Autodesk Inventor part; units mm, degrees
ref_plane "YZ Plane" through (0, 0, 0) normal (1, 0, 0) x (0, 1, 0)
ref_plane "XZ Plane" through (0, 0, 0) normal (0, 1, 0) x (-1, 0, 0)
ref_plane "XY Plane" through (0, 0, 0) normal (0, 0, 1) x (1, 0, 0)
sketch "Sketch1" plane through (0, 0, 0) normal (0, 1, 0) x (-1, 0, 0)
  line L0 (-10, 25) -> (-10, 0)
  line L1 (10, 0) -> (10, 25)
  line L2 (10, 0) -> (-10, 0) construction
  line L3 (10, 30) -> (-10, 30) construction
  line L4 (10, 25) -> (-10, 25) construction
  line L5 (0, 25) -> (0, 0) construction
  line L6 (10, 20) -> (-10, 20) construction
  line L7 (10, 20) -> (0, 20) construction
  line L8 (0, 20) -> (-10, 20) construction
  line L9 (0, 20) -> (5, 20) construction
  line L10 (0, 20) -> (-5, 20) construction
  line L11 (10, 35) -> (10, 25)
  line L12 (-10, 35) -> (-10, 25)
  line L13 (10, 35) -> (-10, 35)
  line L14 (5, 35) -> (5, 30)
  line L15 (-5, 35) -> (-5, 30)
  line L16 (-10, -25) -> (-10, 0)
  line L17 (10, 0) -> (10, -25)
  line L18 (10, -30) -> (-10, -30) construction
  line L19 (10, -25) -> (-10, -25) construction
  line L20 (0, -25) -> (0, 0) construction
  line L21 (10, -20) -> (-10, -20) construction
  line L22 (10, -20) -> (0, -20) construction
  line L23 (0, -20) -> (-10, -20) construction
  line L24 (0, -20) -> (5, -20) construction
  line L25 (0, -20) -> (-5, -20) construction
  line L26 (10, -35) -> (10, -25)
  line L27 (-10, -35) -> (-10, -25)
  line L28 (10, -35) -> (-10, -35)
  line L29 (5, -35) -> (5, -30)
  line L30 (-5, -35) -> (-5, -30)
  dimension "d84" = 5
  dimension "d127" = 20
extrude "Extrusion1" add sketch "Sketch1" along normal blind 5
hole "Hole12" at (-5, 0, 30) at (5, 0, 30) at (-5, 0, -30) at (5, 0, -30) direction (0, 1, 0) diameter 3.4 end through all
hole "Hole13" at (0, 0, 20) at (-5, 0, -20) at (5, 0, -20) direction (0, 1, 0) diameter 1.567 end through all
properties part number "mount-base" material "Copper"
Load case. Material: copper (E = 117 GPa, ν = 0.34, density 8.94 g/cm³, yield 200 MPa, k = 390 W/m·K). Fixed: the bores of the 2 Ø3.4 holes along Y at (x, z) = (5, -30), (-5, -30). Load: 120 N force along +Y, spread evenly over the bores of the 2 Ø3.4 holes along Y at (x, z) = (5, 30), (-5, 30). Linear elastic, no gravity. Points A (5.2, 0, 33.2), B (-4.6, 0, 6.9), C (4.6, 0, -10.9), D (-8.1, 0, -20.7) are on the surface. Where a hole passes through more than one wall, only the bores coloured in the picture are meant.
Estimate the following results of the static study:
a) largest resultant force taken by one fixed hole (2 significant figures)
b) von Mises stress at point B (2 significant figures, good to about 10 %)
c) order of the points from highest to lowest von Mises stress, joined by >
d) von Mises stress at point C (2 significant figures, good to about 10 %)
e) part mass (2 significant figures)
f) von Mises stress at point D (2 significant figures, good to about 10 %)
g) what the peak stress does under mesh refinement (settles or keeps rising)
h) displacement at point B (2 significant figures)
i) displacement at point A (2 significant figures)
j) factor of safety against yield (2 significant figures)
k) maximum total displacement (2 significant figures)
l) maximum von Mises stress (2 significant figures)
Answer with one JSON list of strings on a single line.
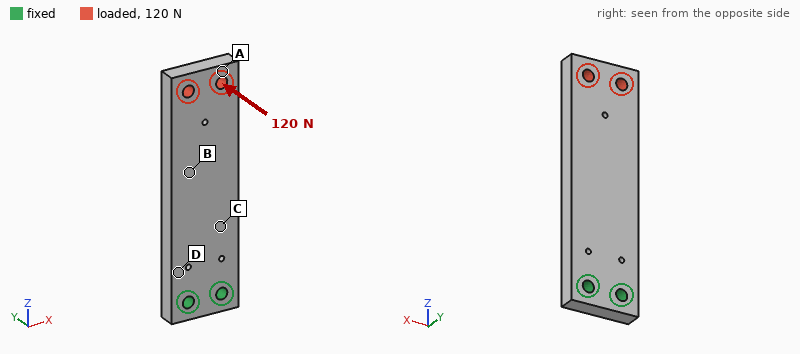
["60 N", "33 MPa", "D > C > B > A", "58 MPa", "61 g", "78 MPa", "settles", "0.16 mm", "0.38 mm", "1.2", "0.39 mm", "160 MPa"]
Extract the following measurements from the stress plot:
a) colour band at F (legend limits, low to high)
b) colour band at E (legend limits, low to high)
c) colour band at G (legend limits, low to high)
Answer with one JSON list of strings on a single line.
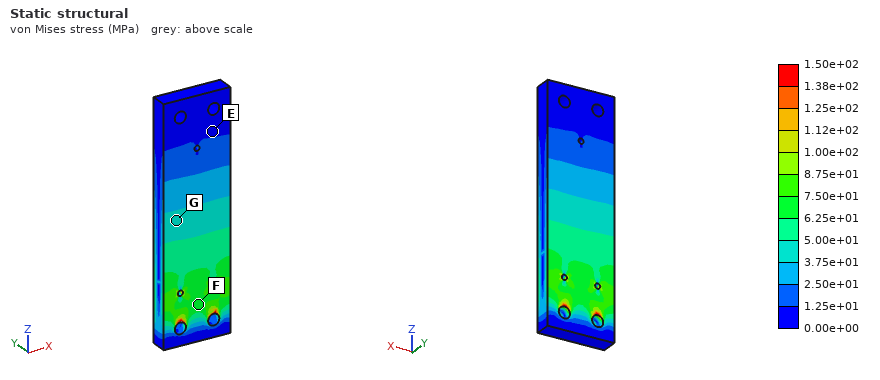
["6.25e+01 to 7.50e+01 MPa", "0.00e+00 to 1.25e+01 MPa", "3.75e+01 to 5.00e+01 MPa"]
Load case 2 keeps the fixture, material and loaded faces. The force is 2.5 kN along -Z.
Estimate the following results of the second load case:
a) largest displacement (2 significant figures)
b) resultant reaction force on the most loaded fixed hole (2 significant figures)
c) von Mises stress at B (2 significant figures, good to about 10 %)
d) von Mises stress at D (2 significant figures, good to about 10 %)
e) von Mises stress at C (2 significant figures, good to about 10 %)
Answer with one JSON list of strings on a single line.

["14 µm", "1.3 kN", "25 MPa", "24 MPa", "25 MPa"]
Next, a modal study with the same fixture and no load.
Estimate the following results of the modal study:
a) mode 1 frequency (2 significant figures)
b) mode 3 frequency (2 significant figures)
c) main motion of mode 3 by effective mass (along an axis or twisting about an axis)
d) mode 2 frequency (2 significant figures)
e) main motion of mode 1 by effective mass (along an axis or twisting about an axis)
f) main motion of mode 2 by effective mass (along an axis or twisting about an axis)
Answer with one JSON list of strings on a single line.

["720 Hz", "4100 Hz", "twisting about Z", "2500 Hz", "along Y", "along X"]
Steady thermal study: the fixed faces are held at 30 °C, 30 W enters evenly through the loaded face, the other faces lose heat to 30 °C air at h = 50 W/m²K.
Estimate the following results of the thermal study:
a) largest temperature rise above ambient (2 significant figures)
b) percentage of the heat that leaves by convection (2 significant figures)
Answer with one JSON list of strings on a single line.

["44 K", "13 %"]
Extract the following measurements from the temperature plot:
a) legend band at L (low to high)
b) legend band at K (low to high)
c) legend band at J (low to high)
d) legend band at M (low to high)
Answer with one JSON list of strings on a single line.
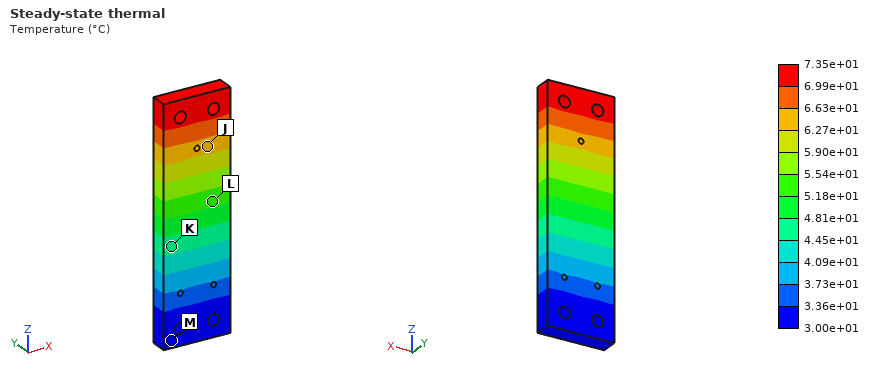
["5.18e+01 to 5.54e+01 °C", "4.45e+01 to 4.81e+01 °C", "6.27e+01 to 6.63e+01 °C", "3.00e+01 to 3.36e+01 °C"]
